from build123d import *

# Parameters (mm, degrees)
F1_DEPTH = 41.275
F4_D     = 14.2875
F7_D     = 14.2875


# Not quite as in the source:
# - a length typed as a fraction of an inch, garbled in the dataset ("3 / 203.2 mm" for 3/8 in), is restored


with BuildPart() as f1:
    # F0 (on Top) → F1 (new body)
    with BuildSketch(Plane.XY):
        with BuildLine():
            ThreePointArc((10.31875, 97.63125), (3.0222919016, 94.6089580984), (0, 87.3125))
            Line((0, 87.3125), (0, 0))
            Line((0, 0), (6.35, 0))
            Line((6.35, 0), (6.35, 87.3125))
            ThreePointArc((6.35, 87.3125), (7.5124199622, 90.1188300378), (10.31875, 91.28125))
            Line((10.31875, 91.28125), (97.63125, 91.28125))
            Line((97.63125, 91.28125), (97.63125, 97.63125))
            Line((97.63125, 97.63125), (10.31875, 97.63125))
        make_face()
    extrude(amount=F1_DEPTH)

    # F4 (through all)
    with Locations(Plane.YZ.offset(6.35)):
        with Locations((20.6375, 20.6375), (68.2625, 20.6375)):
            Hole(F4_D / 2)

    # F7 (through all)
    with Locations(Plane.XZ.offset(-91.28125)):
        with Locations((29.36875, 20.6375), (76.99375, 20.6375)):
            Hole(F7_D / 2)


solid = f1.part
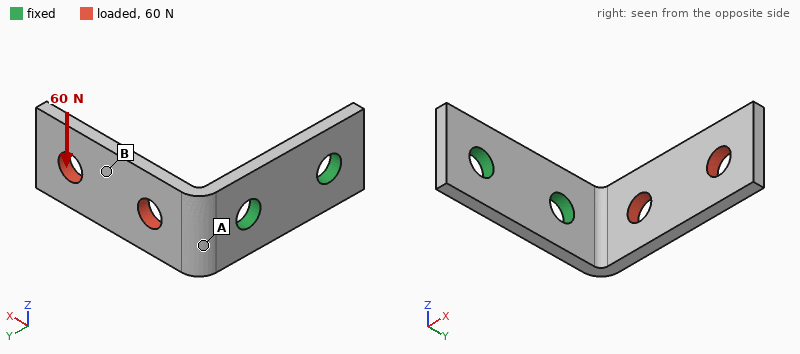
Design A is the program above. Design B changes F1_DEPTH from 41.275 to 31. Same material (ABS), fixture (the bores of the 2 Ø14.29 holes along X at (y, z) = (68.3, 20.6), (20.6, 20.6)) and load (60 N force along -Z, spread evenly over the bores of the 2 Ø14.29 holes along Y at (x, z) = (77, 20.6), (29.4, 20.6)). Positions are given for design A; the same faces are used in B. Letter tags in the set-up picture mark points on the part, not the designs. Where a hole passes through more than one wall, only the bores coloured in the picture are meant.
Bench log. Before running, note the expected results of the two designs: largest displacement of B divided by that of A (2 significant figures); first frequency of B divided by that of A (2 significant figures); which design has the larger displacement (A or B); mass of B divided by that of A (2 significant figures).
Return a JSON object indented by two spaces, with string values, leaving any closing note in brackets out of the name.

{
  "largest displacement of B divided by that of A": "1.5",
  "first frequency of B divided by that of A": "0.99",
  "which design has the larger displacement": "B",
  "mass of B divided by that of A": "0.73"
}
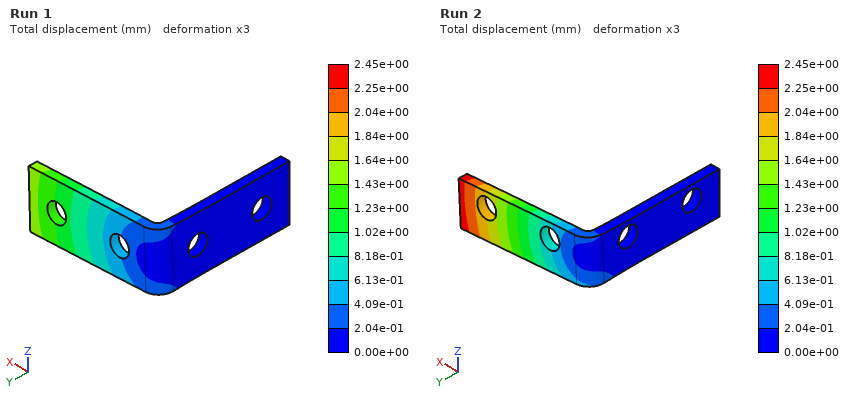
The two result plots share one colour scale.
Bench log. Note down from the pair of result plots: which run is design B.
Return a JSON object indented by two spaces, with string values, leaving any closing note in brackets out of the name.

{
  "which run is design B": "Run 2"
}
